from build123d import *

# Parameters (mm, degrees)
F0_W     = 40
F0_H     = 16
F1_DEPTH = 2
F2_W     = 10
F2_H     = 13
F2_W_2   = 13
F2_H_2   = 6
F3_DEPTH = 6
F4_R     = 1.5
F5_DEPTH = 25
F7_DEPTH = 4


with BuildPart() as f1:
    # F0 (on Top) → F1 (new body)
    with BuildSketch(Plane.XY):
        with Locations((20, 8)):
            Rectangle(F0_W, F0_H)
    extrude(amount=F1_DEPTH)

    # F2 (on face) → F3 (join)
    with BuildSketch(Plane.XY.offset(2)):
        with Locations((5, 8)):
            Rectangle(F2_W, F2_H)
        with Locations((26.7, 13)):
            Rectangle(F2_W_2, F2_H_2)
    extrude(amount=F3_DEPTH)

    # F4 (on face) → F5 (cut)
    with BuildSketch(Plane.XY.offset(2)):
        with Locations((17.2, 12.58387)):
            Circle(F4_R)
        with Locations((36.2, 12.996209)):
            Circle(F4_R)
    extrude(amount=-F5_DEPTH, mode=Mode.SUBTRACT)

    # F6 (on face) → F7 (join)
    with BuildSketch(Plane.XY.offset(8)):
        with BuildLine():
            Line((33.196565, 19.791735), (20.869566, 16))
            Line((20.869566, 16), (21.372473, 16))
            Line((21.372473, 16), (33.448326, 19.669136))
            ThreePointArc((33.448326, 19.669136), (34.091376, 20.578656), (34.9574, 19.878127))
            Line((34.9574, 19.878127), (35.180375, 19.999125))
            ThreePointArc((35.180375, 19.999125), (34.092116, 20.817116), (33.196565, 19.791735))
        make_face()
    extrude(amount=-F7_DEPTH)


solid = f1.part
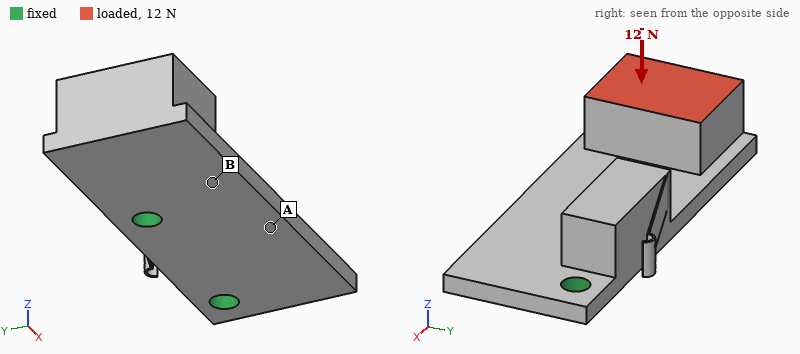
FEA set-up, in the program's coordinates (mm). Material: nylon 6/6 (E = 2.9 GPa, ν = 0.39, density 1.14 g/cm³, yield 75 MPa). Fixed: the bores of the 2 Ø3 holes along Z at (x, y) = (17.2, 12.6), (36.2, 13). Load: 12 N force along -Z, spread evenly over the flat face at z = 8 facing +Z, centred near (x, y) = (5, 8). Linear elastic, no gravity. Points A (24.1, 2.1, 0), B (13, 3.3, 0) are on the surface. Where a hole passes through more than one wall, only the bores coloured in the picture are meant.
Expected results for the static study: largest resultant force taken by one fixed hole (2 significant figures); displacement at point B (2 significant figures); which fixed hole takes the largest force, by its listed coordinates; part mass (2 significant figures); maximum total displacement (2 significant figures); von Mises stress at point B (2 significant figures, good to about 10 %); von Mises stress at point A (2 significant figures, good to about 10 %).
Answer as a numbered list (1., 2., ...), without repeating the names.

1. 14 N
2. 0.100 mm
3. (17.2, 12.6)
4. 2.9 g
5. 0.48 mm
6. 5.9 MPa
7. 2.5 MPa
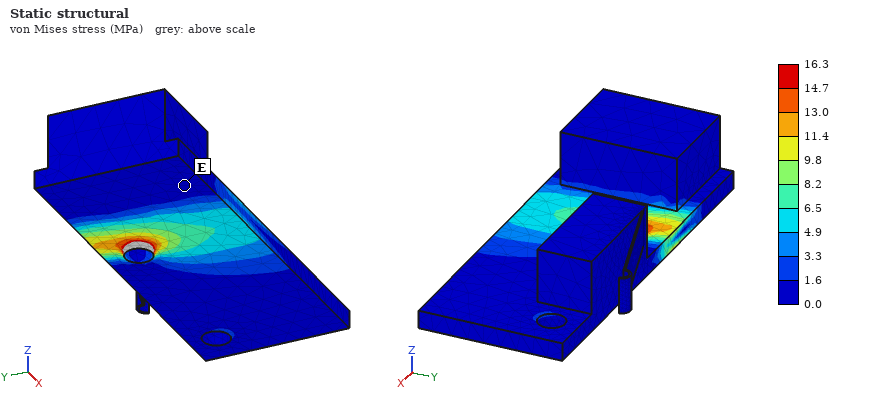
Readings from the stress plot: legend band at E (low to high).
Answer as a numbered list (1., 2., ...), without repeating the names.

1. 0.0 to 1.6 MPa
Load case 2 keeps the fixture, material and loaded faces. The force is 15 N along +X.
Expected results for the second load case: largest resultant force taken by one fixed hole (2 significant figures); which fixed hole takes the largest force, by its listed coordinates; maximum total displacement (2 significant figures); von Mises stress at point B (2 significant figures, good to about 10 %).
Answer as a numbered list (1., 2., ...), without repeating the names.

1. 11 N
2. (17.2, 12.6)
3. 0.43 mm
4. 7.0 MPa
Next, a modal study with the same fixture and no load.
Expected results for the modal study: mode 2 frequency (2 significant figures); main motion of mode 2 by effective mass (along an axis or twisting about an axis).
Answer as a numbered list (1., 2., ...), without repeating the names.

1. 860 Hz
2. along Z
